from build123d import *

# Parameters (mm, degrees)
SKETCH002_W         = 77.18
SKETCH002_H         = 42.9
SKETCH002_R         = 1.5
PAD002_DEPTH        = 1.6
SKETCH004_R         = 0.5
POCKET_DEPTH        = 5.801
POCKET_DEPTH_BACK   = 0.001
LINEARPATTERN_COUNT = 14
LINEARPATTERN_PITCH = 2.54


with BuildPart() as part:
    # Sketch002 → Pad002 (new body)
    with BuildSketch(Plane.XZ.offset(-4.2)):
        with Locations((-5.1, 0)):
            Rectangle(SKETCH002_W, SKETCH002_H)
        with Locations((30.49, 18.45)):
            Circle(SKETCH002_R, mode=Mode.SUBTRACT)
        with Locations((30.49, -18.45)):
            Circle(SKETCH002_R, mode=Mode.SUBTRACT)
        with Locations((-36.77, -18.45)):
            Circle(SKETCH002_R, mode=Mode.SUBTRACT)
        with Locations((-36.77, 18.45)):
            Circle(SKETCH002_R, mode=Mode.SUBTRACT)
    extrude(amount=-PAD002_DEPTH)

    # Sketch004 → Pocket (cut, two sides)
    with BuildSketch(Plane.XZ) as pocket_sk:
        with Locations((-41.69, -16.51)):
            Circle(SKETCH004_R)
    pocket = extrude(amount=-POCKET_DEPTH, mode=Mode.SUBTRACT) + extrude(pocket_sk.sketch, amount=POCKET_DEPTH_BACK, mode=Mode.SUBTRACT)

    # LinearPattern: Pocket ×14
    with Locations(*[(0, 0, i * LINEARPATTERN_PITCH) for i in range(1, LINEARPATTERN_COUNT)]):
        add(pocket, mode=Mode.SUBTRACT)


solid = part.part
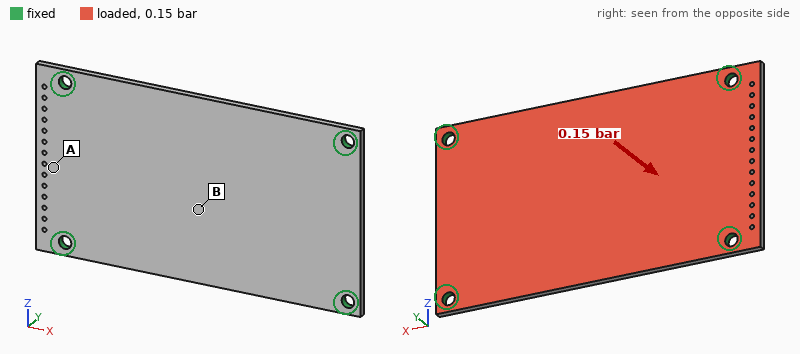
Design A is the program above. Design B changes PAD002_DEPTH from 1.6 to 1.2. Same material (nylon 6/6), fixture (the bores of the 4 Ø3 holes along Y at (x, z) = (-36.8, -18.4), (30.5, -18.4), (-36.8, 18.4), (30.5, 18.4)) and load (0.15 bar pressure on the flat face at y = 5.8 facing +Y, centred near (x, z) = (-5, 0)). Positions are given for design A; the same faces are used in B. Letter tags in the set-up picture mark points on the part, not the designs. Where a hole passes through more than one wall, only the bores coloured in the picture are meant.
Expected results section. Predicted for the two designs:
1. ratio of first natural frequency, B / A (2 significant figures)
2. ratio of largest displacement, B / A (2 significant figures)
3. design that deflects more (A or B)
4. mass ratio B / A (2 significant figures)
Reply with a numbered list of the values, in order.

1. 0.76
2. 2.3
3. B
4. 0.75
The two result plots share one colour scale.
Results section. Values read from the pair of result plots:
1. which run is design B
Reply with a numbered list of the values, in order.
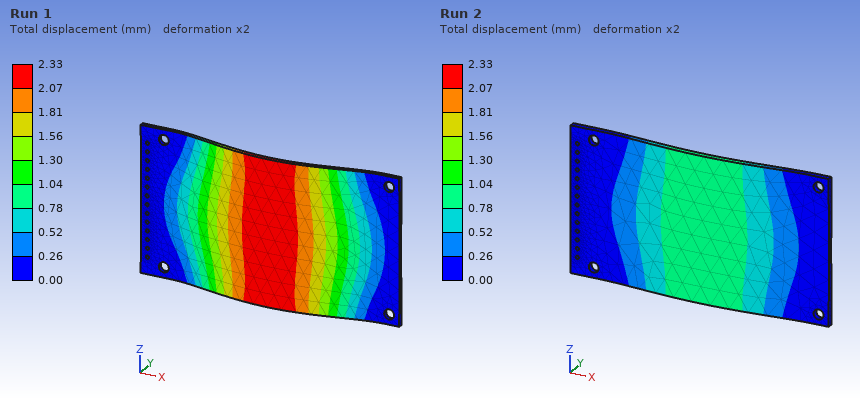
1. Run 1
